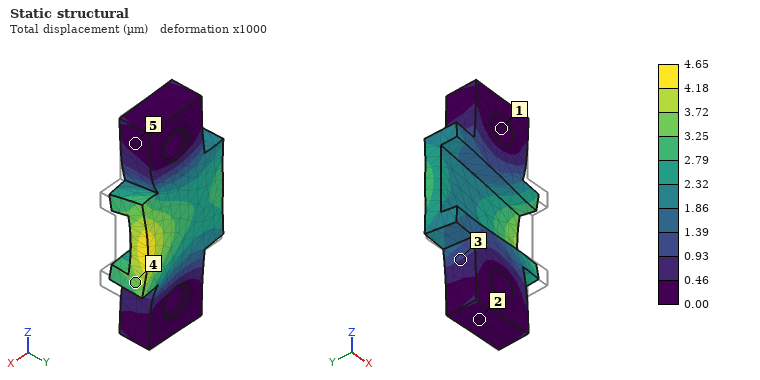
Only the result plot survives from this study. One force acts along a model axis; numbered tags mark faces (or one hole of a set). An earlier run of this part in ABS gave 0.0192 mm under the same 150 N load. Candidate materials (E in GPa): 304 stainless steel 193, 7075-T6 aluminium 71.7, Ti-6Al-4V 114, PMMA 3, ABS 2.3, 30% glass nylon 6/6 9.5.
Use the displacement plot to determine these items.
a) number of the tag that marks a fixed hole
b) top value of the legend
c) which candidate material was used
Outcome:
1
4.65 µm
30% glass nylon 6/6
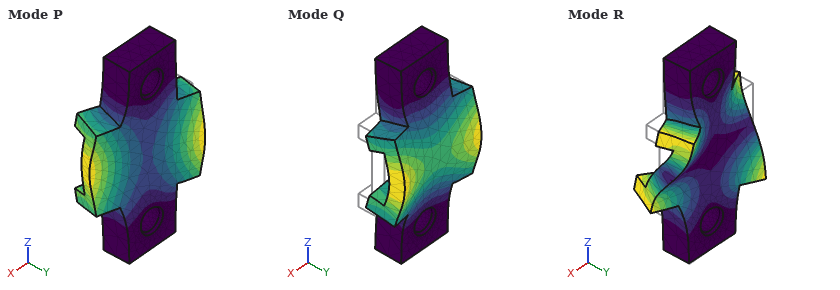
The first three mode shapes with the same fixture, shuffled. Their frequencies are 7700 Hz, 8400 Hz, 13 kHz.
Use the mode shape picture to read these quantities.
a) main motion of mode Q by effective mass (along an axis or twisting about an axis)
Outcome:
along Y
